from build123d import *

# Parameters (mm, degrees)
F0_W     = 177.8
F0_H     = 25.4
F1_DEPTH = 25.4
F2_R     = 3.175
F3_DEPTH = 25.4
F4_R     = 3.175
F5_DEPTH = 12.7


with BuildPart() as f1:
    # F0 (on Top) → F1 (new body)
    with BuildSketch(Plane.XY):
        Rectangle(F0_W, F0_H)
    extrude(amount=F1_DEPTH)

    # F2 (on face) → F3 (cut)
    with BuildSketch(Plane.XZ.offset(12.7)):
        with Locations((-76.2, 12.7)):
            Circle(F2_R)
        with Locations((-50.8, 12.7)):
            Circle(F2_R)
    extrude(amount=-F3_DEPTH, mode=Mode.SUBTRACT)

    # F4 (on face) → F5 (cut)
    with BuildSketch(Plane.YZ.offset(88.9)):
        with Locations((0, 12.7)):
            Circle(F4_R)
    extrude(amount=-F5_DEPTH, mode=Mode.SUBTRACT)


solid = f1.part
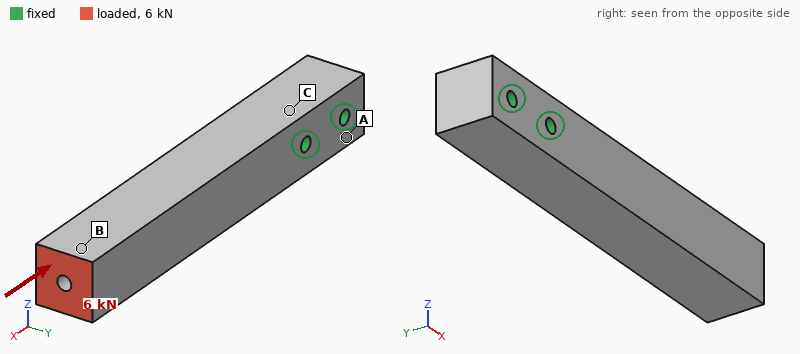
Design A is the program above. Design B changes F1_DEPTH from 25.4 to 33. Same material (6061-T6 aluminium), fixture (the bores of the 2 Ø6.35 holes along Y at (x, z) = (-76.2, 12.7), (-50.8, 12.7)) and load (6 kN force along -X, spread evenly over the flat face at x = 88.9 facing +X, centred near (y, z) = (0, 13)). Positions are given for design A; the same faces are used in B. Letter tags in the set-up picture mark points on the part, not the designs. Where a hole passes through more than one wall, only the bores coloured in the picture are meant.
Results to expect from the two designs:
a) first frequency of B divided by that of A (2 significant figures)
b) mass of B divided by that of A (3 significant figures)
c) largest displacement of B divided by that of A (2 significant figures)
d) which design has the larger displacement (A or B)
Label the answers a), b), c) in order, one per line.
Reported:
a) 1.1
b) 1.30
c) 1.1
d) B
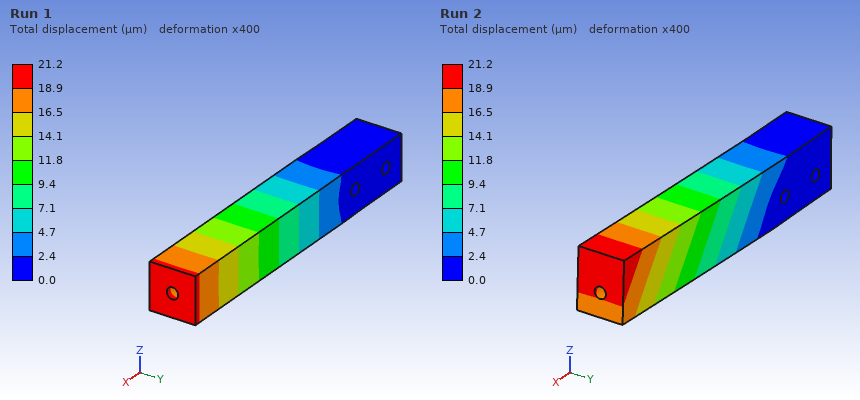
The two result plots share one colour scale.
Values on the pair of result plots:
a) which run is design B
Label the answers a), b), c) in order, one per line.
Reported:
a) Run 2
